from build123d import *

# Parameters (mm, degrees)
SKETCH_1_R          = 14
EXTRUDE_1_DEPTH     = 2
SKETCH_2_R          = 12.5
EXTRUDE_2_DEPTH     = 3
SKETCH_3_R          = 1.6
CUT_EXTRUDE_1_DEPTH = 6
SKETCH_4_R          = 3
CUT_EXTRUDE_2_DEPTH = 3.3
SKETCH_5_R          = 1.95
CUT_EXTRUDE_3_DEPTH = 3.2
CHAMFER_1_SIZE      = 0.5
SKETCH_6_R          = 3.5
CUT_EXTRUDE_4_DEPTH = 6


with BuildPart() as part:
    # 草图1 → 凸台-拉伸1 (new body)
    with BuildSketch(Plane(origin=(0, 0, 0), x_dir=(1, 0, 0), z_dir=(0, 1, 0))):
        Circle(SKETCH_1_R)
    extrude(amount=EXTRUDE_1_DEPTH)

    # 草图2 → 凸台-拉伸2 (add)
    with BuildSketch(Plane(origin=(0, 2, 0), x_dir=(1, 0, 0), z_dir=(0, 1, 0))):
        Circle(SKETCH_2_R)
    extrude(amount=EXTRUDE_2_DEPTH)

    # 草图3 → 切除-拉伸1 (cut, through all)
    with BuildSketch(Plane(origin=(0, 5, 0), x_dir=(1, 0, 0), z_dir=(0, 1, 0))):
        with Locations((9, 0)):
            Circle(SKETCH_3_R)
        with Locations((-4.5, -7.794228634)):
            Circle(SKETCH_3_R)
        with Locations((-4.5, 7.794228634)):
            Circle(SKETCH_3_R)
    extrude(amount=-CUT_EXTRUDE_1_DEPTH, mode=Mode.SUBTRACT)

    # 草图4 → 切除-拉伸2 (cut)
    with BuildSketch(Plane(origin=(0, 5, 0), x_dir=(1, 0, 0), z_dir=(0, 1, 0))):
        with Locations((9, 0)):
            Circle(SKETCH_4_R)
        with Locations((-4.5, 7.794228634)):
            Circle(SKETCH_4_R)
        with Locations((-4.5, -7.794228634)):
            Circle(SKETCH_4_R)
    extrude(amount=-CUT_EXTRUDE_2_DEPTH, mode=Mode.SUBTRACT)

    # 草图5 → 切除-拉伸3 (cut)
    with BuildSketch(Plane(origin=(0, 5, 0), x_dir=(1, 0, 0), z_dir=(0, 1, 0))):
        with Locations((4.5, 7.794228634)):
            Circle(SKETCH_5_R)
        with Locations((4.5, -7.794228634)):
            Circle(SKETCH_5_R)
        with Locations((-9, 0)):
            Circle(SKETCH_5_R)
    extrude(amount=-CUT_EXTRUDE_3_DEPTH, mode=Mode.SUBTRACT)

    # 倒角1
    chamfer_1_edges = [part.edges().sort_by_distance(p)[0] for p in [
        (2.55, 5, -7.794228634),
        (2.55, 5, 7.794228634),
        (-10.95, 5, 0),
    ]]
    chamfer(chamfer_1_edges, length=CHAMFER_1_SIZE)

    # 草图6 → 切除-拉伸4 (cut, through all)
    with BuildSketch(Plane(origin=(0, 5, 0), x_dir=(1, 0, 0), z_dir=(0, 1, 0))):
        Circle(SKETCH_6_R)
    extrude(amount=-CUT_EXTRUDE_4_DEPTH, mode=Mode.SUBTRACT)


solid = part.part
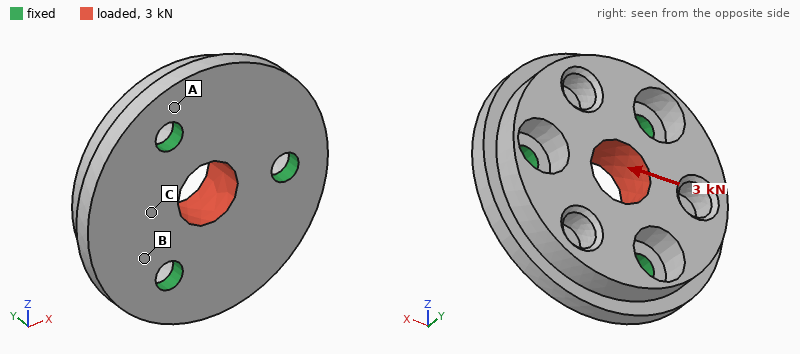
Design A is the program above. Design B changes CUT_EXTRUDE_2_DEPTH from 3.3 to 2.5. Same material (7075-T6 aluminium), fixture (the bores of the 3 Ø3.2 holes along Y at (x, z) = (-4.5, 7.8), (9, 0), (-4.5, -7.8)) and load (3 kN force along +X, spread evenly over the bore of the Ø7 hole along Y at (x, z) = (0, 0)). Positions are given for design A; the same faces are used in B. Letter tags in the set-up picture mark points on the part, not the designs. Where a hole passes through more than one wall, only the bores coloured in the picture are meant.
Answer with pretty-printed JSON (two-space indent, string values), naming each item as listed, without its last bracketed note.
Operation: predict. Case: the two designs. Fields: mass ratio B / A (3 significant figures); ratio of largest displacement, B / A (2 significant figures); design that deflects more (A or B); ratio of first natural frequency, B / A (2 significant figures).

{
  "mass ratio B / A": "1.02",
  "ratio of largest displacement, B / A": "0.60",
  "design that deflects more": "A",
  "ratio of first natural frequency, B / A": "1.2"
}
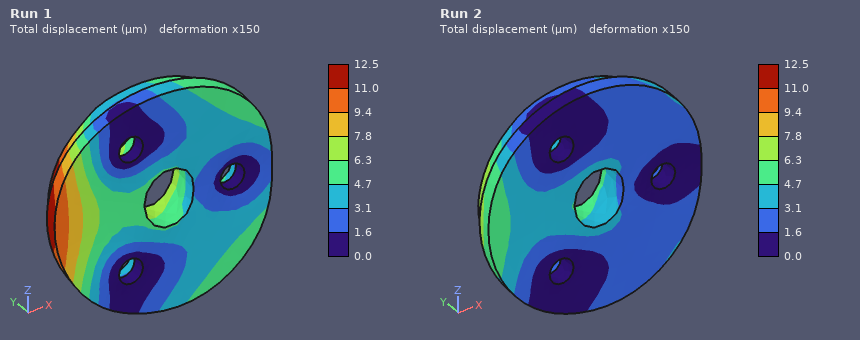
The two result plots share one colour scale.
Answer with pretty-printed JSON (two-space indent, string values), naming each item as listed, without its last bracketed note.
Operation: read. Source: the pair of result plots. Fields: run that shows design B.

{
  "run that shows design B": "Run 2"
}
